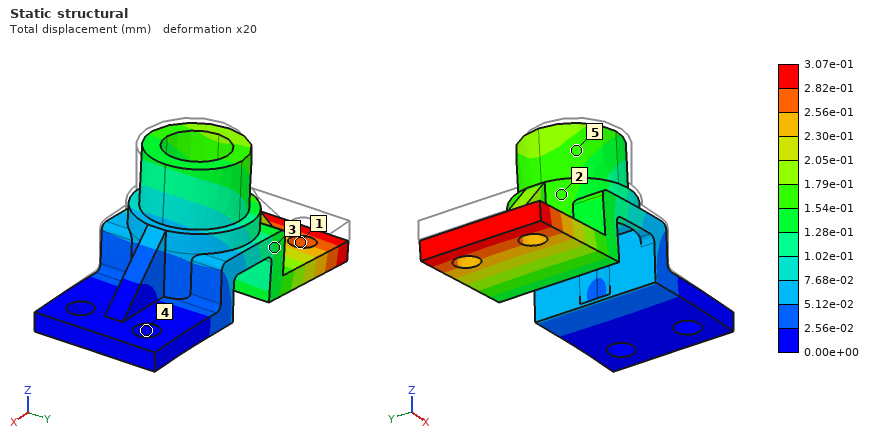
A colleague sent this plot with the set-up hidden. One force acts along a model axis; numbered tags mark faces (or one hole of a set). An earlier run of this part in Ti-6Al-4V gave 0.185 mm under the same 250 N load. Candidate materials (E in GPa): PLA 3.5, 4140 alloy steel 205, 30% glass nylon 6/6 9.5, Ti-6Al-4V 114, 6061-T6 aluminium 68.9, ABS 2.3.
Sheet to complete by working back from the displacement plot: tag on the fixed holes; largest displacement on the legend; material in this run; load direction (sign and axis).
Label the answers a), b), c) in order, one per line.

a) 4
b) 3.07e-01 mm
c) 6061-T6 aluminium
d) -Z
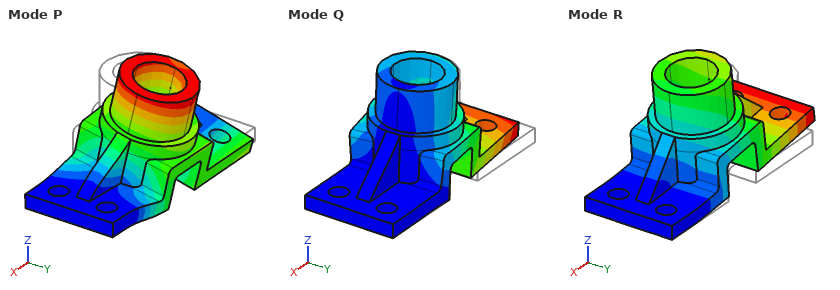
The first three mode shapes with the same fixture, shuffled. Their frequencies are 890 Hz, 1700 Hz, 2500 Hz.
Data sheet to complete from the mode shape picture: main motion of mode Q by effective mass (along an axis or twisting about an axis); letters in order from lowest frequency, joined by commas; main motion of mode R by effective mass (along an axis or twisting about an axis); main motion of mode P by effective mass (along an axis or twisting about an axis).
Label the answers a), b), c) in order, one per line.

a) along Y
b) R, Q, P
c) along Z
d) along Y
